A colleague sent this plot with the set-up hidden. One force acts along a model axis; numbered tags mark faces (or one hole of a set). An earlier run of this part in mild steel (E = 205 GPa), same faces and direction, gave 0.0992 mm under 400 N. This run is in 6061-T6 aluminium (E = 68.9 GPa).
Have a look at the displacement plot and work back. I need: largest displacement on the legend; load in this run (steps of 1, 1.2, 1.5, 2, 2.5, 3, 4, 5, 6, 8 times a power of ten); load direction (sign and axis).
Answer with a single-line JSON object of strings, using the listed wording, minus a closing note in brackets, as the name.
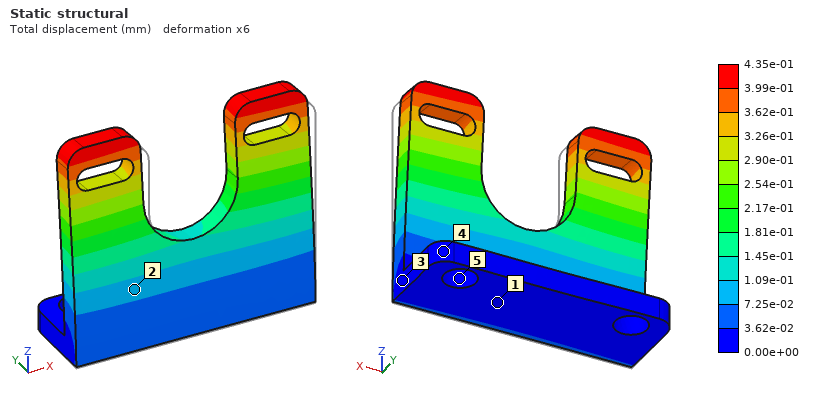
{"largest displacement on the legend": "4.35e-01 mm", "load in this run": "600 N", "load direction": "+Y"}
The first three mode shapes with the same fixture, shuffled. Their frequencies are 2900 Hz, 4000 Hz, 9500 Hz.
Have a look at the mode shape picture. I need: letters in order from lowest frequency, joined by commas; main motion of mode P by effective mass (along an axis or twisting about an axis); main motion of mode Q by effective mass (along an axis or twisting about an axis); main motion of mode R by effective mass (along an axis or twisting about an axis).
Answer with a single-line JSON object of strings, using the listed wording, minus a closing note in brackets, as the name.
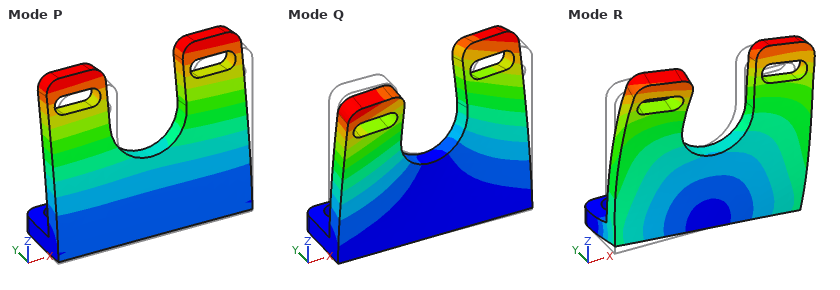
{"letters in order from lowest frequency, joined by commas": "P, Q, R", "main motion of mode P by effective mass": "along Y", "main motion of mode Q by effective mass": "twisting about Z", "main motion of mode R by effective mass": "along X"}
